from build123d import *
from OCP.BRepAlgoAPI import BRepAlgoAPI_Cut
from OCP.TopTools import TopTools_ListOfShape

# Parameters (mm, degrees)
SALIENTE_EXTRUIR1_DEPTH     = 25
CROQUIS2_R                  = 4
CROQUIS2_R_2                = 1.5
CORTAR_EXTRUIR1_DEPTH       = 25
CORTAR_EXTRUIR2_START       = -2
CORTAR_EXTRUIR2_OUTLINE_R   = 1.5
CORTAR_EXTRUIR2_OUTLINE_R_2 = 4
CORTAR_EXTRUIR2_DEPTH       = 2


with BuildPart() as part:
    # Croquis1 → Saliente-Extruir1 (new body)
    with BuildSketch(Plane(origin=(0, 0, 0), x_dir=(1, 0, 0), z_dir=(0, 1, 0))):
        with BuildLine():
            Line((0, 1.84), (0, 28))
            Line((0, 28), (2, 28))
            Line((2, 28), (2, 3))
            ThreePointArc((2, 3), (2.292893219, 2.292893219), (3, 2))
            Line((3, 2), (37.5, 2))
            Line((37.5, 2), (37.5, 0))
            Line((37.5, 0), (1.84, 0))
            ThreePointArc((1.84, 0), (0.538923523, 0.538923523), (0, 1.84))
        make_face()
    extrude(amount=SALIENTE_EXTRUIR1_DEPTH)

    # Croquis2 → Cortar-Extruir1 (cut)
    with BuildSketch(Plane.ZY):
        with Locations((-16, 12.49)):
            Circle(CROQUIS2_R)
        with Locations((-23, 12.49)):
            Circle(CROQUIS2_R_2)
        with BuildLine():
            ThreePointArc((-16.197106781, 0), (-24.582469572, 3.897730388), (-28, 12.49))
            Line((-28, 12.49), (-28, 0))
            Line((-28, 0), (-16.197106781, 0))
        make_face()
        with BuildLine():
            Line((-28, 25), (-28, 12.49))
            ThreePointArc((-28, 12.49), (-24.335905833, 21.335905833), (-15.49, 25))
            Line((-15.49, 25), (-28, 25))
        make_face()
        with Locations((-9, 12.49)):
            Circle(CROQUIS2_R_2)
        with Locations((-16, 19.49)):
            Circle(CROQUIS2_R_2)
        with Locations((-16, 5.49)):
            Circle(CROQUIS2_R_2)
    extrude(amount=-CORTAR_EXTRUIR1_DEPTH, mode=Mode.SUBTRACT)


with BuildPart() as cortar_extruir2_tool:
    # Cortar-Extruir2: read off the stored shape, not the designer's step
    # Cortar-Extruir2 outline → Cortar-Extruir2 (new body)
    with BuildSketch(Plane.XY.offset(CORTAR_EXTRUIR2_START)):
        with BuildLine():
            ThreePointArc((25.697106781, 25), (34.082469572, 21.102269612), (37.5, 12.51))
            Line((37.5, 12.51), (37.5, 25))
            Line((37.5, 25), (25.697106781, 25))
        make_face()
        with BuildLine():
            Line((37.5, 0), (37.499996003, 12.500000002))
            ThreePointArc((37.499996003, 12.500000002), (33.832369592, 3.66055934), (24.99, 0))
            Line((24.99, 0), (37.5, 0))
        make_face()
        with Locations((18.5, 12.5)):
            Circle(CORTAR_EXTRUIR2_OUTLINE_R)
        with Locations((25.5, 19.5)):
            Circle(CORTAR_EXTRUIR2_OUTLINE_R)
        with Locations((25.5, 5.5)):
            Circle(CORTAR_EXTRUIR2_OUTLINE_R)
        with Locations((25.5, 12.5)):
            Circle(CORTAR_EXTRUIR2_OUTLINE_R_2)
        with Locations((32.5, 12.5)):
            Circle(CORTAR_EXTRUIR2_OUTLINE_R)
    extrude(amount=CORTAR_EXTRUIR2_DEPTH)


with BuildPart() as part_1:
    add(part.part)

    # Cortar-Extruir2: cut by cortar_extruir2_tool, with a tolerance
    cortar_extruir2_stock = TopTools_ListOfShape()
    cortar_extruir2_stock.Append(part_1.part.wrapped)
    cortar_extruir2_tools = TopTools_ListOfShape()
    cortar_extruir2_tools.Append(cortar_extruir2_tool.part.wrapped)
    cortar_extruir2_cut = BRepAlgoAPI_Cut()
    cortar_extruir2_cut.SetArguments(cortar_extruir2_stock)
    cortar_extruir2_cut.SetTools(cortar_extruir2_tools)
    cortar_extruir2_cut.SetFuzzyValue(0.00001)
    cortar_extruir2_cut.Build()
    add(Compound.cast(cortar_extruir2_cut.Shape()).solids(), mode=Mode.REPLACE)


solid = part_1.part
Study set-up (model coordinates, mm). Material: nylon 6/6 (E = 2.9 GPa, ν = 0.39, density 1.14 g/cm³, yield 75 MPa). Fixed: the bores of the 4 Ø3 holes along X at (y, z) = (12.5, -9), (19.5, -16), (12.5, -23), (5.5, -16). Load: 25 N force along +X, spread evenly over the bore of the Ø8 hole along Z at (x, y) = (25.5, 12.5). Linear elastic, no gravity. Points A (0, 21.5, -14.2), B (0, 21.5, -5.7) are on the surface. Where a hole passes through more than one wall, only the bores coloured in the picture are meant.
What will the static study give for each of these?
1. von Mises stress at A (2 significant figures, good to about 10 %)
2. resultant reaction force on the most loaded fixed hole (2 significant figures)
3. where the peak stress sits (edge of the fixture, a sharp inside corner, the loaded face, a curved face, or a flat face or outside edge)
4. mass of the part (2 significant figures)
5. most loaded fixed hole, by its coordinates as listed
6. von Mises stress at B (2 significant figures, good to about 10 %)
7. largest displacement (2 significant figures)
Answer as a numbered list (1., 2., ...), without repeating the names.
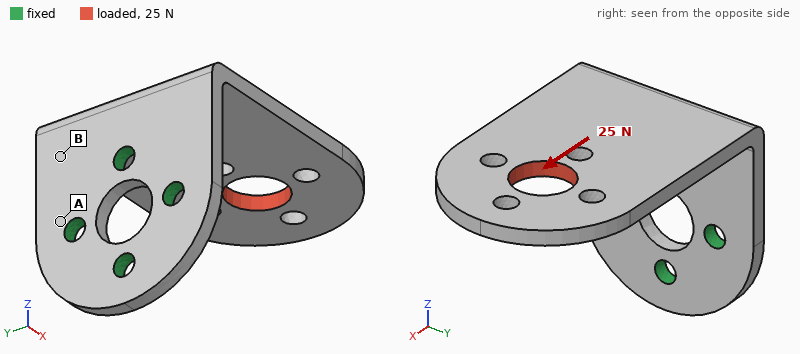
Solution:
1. 1.7 MPa
2. 32 N
3. a flat face or outside edge
4. 2.9 g
5. (12.5, -9)
6. 4.0 MPa
7. 0.63 mm
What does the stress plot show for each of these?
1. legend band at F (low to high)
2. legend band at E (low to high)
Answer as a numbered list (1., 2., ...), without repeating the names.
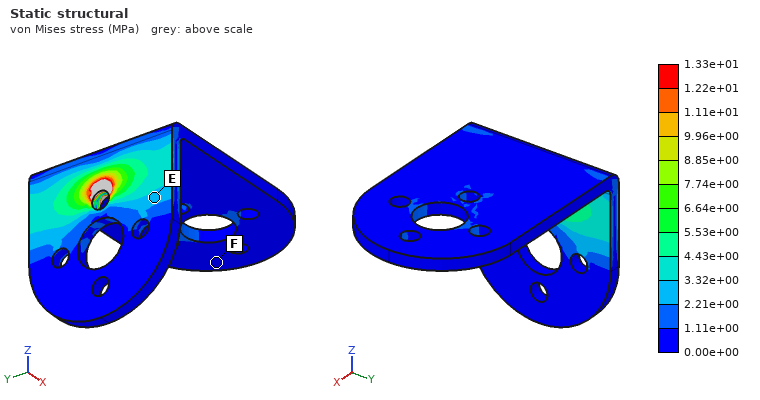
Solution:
1. 0.00e+00 to 1.11e+00 MPa
2. 2.21e+00 to 3.32e+00 MPa
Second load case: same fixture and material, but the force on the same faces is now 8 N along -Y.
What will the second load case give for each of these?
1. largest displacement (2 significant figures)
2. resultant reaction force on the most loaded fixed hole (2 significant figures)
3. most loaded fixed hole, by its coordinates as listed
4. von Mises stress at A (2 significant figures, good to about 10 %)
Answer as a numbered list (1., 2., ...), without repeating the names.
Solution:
1. 0.56 mm
2. 7.7 N
3. (12.5, -9)
4. 7.3 MPa
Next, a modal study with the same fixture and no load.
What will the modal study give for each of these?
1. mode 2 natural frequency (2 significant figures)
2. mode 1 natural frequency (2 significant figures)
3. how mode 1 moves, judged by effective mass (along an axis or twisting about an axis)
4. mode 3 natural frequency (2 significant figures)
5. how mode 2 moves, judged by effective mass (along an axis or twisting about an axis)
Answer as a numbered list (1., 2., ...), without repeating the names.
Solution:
1. 660 Hz
2. 370 Hz
3. along Z
4. 1400 Hz
5. along Y
